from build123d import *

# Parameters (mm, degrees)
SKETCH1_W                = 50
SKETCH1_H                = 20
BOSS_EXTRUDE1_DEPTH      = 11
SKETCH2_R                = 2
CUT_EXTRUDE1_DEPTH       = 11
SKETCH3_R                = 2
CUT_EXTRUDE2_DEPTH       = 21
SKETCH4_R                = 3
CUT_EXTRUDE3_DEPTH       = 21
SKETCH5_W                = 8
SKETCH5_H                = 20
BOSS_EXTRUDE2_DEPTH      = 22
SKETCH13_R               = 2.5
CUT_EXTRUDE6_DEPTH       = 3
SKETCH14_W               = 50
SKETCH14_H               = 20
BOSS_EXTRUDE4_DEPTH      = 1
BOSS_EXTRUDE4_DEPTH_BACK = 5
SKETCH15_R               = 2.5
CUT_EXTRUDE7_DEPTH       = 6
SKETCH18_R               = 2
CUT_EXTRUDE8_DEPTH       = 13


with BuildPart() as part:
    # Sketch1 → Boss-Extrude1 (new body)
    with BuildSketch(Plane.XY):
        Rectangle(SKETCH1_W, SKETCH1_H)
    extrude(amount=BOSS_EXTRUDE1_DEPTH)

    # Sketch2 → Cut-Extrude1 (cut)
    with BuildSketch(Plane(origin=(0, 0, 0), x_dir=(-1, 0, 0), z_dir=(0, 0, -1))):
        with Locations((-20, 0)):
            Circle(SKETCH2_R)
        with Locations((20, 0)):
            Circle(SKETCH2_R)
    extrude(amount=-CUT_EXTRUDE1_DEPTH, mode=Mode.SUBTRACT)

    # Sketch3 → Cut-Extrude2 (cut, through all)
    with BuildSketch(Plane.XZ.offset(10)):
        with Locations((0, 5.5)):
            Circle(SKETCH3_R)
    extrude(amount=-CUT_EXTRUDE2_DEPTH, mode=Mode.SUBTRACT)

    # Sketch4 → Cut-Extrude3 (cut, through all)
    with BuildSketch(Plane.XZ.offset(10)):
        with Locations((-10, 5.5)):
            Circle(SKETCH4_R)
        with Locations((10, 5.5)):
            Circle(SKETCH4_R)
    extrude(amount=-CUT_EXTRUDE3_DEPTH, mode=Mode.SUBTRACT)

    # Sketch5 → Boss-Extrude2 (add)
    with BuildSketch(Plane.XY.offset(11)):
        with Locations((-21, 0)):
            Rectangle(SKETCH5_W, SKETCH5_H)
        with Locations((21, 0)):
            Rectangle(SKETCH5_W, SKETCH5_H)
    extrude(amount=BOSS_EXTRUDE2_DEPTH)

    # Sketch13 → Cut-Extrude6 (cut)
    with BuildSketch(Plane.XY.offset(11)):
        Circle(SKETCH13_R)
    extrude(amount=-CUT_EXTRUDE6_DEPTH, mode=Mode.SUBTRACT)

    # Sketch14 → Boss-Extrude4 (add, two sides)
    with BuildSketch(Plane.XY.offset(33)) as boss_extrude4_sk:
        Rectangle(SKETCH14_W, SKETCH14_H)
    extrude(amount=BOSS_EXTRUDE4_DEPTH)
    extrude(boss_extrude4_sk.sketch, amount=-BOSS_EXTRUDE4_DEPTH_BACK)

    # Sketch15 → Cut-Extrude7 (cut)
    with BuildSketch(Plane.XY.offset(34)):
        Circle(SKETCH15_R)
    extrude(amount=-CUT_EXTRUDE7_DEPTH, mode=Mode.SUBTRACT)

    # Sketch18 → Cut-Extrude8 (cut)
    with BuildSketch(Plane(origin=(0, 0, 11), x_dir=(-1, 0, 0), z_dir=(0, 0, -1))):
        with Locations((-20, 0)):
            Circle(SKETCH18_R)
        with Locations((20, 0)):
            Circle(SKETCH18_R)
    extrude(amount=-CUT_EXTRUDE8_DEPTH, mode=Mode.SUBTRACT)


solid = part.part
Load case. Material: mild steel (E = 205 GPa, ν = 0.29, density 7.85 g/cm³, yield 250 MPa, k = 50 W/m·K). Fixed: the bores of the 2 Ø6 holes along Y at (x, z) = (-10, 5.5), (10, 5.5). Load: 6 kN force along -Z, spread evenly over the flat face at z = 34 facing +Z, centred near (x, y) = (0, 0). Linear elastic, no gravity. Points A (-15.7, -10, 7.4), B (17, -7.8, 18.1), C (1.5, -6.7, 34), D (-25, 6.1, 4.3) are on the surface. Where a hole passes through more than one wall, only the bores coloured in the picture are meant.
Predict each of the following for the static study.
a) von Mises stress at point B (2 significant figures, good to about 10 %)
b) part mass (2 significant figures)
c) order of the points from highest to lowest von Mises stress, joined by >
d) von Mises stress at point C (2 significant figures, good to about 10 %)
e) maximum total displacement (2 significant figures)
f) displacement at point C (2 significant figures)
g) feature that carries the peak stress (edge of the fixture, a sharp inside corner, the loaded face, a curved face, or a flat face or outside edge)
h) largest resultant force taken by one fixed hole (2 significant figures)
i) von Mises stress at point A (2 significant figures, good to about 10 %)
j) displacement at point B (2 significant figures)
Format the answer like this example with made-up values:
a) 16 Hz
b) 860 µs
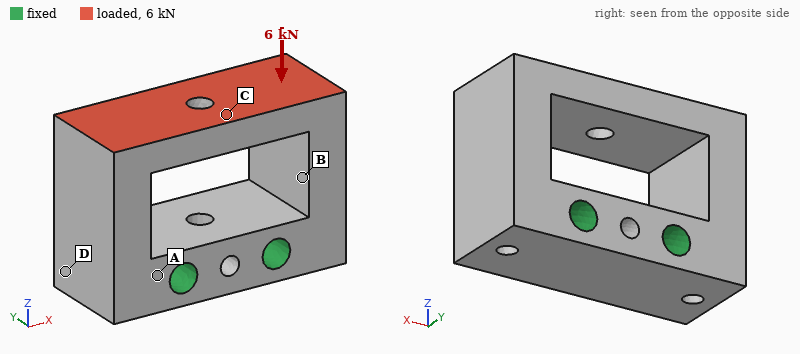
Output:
a) 64 MPa
b) 160 g
c) C > B > A > D
d) 93 MPa
e) 27 µm
f) 26 µm
g) the loaded face
h) 3.0 kN
i) 44 MPa
j) 6.3 µm
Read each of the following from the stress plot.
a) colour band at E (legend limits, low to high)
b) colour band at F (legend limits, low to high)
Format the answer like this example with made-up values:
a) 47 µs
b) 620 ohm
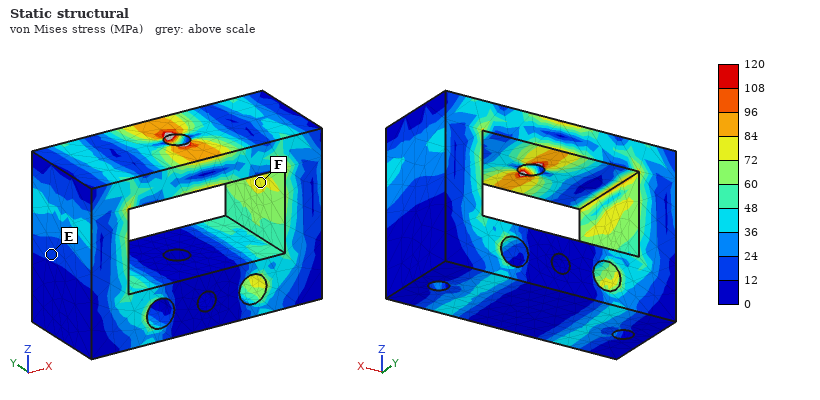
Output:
a) 12 to 24 MPa
b) 72 to 84 MPa
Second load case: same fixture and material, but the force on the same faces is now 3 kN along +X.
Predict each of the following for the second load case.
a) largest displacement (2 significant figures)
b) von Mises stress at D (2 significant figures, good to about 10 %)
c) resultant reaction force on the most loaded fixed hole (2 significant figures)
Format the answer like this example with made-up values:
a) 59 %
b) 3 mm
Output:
a) 41 µm
b) 22 MPa
c) 1.9 kN
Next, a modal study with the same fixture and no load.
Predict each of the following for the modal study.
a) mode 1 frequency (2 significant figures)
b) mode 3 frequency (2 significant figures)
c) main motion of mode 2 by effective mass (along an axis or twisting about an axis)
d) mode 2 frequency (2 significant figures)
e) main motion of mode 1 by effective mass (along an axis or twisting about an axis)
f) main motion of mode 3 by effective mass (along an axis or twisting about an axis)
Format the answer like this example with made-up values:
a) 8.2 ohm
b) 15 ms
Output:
a) 6000 Hz
b) 11 kHz
c) along Y
d) 7100 Hz
e) along X
f) twisting about Z
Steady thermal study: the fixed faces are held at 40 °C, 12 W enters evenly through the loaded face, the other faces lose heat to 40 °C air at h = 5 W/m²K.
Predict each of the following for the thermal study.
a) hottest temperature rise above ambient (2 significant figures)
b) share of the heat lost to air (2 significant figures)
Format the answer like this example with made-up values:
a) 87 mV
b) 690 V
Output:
a) 29 K
b) 3.1 %
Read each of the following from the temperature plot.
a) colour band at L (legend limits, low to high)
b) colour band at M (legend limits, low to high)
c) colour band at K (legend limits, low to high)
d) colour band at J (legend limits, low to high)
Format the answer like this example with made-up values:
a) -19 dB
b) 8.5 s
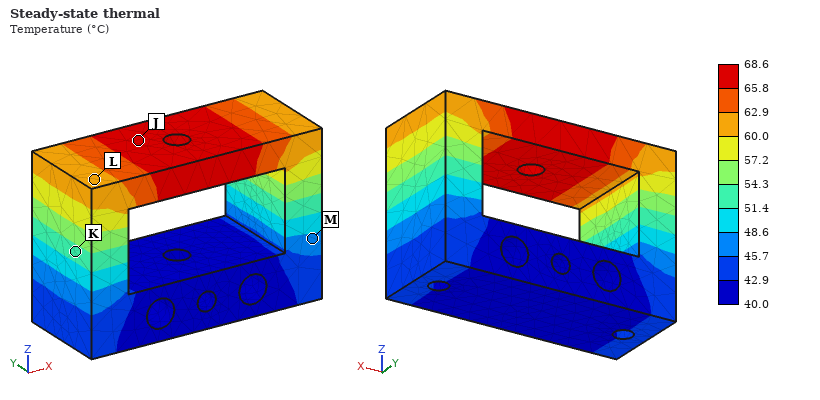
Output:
a) 60.0 to 62.9 °C
b) 45.7 to 48.6 °C
c) 51.4 to 54.3 °C
d) 65.8 to 68.6 °C
